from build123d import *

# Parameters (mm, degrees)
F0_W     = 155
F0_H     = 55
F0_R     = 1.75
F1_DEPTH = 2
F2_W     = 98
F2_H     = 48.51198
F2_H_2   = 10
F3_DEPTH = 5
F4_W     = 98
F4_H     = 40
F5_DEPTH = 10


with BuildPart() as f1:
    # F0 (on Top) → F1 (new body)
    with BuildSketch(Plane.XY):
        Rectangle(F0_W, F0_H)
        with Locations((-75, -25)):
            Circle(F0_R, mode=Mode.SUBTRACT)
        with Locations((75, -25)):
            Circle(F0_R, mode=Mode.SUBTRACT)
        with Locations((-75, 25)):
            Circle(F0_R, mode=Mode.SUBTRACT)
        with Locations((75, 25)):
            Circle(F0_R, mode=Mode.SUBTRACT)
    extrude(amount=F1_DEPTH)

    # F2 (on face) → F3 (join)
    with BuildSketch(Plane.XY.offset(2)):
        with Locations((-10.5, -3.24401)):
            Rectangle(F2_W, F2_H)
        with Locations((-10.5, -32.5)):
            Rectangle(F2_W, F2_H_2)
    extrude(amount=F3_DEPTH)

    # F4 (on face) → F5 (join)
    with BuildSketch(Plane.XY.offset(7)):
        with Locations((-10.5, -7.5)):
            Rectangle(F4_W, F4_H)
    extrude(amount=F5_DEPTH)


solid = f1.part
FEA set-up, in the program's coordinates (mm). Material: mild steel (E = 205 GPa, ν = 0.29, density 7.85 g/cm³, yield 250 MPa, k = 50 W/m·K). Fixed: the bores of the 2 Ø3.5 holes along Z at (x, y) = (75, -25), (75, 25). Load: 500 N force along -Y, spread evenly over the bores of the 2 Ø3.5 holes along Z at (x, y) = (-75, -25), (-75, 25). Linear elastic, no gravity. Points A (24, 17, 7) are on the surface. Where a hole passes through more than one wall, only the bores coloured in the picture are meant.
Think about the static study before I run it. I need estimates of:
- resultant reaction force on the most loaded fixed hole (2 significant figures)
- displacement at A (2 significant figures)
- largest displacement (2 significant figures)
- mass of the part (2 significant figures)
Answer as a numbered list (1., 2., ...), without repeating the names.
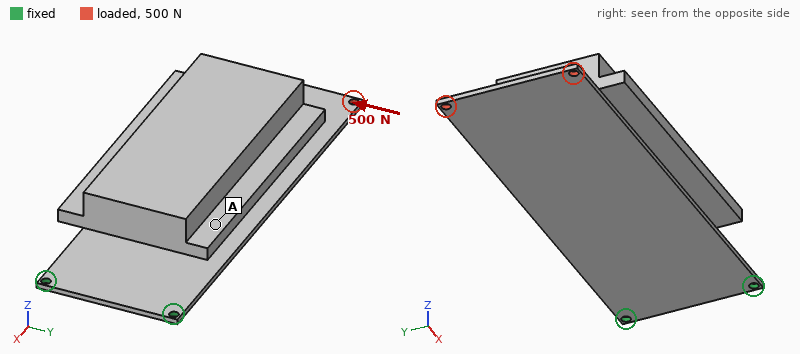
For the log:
1. 1.5 kN
2. 22 µm
3. 92 µm
4. 670 g
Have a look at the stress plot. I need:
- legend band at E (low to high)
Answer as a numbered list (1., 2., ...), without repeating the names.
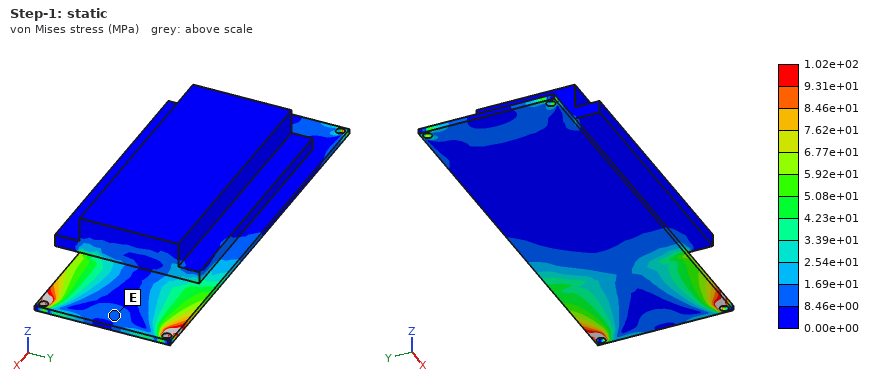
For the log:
1. 8.46e+00 to 1.69e+01 MPa
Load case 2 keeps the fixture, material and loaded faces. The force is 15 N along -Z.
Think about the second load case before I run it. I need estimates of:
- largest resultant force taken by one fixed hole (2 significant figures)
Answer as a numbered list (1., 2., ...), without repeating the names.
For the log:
1. 8.0 N
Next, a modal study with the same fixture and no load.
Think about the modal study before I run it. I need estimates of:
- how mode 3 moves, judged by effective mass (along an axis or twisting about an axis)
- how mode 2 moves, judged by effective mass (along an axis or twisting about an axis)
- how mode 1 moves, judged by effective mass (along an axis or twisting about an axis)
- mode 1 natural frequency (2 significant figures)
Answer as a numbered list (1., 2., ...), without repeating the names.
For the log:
1. along Z
2. along Y
3. along Z
4. 33 Hz
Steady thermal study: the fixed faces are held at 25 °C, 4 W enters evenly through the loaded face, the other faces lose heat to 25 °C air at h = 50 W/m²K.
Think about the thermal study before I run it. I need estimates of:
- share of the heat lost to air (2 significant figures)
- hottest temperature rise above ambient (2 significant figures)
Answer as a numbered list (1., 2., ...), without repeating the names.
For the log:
1. 97 %
2. 36 K
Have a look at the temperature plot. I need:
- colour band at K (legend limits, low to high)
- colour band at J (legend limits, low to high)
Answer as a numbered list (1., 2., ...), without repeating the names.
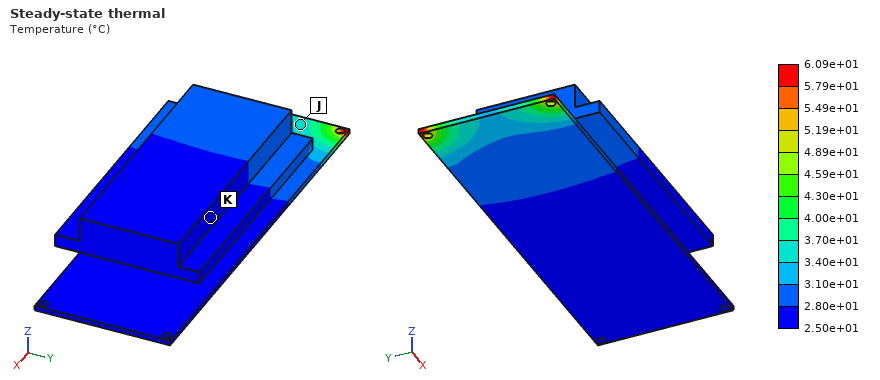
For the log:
1. 2.50e+01 to 2.80e+01 °C
2. 3.40e+01 to 3.70e+01 °C
